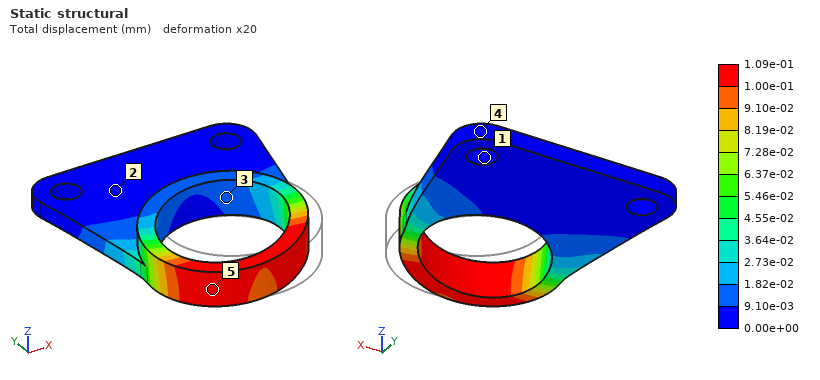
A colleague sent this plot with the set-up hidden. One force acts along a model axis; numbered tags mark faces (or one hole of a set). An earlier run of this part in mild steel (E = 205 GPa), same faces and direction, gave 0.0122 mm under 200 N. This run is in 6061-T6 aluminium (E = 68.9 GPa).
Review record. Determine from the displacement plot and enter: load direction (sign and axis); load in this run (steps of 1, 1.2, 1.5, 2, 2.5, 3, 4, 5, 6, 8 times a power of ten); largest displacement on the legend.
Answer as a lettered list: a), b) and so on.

a) -X
b) 600 N
c) 1.09e-01 mm
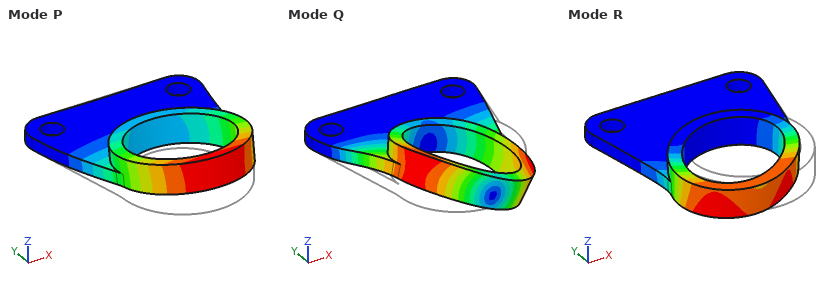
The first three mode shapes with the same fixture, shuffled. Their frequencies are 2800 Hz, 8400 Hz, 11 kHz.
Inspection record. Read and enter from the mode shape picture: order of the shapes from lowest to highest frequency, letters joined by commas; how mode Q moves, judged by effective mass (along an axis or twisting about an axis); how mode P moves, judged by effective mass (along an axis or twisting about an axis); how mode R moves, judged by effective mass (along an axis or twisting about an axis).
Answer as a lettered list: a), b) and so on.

a) P, Q, R
b) twisting about Y
c) along Z
d) along X
